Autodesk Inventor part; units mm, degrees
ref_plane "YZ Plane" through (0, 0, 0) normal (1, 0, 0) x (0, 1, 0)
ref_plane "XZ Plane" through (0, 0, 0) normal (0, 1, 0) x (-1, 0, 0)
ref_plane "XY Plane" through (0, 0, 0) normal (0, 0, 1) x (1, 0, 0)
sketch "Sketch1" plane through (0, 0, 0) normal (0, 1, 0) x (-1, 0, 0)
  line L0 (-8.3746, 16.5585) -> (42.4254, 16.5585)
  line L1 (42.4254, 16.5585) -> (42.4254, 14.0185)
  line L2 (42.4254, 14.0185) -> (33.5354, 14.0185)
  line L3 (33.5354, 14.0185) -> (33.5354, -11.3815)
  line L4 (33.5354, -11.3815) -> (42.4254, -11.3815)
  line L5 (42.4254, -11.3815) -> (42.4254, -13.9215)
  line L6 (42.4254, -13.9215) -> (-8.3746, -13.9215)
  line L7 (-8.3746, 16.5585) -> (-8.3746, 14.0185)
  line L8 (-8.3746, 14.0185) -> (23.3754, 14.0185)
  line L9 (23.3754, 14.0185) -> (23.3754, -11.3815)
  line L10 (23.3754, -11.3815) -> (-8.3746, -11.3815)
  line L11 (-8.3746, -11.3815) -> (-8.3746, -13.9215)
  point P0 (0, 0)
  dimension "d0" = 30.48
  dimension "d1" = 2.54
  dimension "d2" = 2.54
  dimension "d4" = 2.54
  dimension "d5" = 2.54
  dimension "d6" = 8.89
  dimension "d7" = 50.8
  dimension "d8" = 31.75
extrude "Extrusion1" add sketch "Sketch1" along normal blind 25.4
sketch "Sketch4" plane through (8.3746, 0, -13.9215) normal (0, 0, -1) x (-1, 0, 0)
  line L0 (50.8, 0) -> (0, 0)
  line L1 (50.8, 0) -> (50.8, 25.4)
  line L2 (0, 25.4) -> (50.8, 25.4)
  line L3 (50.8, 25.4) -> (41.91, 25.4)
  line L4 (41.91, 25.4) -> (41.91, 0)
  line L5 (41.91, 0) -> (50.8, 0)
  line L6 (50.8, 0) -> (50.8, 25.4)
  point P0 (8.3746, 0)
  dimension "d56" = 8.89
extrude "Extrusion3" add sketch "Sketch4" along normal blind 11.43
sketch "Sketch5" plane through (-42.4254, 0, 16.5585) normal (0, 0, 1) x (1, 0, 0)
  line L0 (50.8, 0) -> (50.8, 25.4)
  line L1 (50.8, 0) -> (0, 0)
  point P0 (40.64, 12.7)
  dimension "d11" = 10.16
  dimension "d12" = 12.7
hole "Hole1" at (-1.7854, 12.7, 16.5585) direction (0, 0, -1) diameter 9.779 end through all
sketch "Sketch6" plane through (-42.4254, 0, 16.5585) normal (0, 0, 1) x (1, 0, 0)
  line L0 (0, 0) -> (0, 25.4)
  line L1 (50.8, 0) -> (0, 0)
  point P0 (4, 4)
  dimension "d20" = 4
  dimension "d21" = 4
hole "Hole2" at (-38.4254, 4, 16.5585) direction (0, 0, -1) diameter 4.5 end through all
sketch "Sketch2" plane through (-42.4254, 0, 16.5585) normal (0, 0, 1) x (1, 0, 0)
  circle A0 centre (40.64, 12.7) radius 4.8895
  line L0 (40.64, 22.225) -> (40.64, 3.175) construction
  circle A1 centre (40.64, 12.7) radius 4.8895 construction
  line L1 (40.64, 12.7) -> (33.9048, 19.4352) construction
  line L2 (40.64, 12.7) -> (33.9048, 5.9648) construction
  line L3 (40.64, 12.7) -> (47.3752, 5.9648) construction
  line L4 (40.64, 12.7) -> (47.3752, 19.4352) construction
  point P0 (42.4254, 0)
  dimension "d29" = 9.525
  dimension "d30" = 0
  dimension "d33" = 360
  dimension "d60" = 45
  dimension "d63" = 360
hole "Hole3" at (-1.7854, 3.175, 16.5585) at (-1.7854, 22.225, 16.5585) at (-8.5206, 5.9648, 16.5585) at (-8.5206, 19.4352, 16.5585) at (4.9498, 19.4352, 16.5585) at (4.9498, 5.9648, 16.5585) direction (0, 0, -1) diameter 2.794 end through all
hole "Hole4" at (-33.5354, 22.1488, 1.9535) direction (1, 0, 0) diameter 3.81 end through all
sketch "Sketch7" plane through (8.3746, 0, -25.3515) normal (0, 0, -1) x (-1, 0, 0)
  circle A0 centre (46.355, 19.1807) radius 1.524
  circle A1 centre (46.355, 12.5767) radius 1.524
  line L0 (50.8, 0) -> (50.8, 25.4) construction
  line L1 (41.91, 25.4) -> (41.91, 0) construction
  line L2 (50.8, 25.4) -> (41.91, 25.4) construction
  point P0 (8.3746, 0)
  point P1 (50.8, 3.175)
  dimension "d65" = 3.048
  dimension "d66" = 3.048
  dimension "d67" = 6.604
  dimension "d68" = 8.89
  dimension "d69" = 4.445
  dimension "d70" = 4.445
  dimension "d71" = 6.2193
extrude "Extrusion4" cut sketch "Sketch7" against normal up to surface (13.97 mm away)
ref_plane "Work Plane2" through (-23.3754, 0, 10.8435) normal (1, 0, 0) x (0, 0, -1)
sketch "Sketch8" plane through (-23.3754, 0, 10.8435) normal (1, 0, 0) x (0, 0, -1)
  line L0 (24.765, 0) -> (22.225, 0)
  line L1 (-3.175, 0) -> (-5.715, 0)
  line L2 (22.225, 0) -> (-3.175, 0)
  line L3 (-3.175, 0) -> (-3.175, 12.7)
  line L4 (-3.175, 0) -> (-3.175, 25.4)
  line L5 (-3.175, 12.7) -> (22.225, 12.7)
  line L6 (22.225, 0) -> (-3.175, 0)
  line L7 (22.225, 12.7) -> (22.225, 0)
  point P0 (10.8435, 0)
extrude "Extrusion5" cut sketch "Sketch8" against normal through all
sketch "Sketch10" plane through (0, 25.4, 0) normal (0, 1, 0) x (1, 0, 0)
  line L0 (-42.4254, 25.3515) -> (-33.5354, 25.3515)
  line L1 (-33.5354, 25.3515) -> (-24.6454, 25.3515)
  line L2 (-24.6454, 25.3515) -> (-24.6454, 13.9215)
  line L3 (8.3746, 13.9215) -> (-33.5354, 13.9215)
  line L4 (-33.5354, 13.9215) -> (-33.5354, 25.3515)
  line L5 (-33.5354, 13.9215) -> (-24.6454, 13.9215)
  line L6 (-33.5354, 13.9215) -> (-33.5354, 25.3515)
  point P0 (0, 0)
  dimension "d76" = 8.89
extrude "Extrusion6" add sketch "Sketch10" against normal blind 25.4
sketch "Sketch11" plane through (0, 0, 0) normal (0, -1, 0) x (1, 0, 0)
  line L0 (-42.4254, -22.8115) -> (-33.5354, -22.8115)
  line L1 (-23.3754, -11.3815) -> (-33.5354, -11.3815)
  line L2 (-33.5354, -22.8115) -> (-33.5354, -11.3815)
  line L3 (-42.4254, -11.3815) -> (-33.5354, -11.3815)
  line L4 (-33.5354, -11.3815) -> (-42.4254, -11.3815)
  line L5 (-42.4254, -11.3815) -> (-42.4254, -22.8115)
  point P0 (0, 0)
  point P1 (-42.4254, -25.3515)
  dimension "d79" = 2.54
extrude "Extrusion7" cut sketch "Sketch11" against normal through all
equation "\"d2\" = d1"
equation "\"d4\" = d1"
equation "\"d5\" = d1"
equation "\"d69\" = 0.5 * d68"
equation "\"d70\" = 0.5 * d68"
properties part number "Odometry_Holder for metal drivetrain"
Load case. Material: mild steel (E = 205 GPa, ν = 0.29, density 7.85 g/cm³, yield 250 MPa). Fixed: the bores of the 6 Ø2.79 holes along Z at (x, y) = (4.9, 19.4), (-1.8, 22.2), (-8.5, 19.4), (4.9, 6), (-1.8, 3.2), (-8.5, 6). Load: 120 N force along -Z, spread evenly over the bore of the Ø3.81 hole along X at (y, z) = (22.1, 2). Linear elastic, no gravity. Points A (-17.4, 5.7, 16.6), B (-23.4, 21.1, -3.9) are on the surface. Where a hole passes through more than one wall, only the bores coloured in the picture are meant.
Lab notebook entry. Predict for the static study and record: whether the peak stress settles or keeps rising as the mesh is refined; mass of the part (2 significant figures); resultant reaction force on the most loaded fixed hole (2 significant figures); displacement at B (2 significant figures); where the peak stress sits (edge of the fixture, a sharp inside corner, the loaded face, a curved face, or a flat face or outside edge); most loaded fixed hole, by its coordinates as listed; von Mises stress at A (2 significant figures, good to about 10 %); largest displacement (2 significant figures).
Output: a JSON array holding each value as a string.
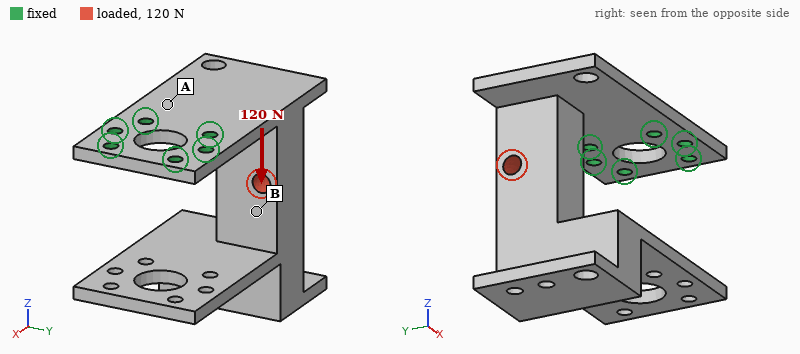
["keeps rising", "91 g", "180 N", "0.073 mm", "edge of the fixture", "(-8.5, 19.4)", "46 MPa", "0.17 mm"]
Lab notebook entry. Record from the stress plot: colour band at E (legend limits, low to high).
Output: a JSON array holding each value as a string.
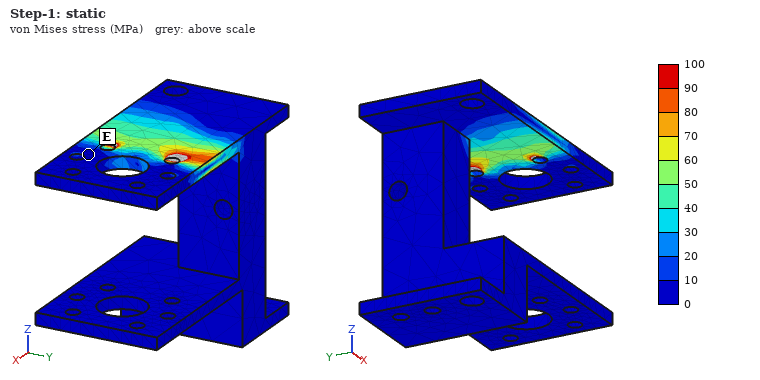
["0 to 10 MPa"]
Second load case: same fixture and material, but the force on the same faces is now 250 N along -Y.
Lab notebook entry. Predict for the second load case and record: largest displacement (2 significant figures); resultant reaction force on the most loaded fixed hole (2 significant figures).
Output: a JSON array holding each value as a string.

["0.14 mm", "350 N"]
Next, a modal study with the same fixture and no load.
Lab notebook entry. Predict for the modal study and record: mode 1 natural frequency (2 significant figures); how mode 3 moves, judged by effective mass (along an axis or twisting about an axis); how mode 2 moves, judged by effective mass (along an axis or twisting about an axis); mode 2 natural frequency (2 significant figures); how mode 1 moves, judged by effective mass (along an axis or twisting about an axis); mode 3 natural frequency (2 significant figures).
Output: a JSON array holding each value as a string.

["400 Hz", "along Z", "along Y", "680 Hz", "along X", "1800 Hz"]
